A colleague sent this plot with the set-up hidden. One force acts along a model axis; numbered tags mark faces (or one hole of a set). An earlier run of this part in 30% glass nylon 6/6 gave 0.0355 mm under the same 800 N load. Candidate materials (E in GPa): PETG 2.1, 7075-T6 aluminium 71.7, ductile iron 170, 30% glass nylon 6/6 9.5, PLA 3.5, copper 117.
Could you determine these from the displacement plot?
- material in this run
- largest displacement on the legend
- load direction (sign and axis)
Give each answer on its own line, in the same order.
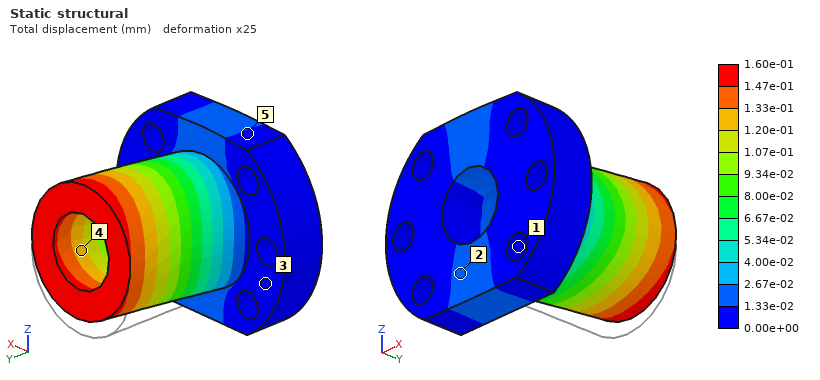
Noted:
PETG
1.60e-01 mm
+Z
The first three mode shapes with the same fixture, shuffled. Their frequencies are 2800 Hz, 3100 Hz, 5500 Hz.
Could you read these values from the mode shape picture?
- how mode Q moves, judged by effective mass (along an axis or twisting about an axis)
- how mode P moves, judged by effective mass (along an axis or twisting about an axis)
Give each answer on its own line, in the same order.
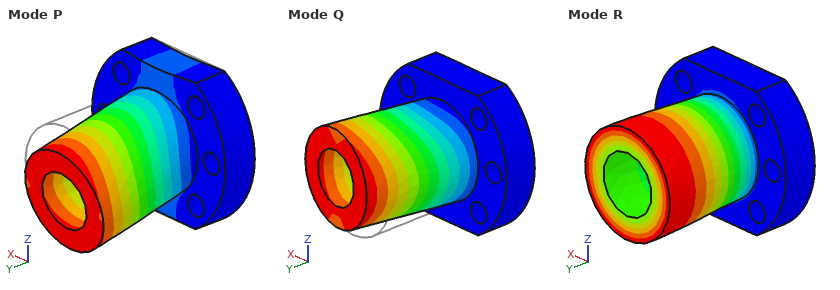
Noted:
along X
along Z
